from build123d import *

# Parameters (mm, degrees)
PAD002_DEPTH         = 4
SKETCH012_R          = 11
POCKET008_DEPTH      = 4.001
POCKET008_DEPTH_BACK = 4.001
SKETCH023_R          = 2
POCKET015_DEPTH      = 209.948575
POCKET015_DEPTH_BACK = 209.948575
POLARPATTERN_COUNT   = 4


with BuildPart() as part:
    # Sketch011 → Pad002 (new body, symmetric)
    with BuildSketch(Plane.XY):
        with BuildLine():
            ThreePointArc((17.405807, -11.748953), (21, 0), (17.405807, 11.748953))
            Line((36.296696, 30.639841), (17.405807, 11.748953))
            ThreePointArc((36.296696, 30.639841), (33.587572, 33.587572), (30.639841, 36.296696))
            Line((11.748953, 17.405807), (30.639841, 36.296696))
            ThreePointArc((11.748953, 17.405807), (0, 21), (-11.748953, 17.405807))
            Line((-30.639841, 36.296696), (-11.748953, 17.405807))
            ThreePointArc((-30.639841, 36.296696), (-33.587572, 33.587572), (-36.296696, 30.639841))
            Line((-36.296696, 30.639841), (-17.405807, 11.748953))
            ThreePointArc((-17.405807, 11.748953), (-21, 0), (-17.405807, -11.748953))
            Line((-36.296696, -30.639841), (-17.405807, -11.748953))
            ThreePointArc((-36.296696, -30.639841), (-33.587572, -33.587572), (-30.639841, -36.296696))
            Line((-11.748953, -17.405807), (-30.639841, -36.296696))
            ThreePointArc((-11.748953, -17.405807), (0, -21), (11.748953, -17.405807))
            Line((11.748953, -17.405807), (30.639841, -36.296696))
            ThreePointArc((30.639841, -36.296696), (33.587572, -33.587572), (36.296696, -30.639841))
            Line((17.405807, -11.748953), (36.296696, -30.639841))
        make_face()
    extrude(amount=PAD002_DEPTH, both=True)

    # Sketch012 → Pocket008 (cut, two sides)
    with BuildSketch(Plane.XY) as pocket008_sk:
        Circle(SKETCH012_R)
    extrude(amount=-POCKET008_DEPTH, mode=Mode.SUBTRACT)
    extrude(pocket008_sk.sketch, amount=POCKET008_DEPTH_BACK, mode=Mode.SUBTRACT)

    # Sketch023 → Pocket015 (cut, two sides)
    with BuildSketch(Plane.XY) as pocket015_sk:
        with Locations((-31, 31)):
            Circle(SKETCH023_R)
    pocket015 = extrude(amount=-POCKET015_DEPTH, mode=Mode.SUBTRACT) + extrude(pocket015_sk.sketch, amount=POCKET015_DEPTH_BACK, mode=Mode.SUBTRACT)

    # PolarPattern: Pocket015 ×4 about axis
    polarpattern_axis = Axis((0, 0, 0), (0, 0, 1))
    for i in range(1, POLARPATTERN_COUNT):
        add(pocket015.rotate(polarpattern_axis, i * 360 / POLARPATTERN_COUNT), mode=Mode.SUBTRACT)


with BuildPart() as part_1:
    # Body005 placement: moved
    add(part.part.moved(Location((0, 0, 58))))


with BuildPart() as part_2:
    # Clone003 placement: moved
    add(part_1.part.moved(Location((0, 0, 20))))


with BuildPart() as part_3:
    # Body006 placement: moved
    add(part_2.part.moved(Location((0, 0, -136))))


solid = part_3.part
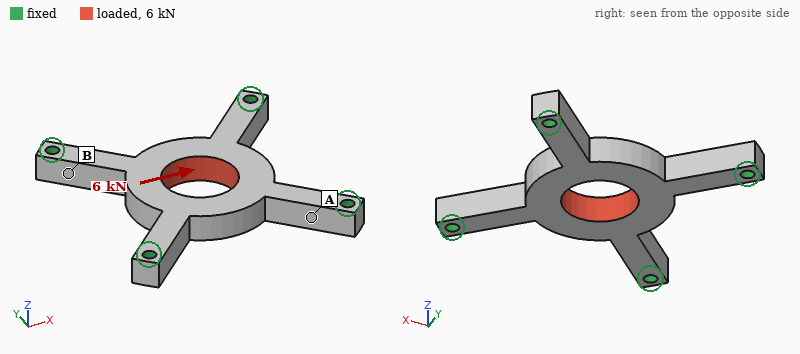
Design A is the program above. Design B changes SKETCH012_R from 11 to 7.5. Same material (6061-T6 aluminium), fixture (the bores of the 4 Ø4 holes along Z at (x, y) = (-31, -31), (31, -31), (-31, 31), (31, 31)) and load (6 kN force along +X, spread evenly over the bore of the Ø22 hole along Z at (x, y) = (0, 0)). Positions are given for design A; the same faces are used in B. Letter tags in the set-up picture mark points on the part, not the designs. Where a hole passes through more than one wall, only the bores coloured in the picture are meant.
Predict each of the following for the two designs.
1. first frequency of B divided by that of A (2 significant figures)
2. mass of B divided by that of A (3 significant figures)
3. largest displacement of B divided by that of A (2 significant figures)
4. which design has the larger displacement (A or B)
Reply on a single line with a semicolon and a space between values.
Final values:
0.95; 1.11; 0.87; A
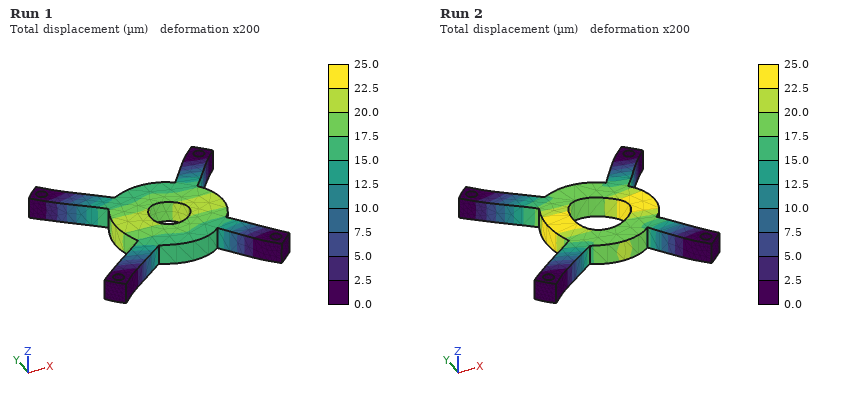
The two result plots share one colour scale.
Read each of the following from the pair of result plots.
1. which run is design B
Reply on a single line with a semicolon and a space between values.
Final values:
Run 1
